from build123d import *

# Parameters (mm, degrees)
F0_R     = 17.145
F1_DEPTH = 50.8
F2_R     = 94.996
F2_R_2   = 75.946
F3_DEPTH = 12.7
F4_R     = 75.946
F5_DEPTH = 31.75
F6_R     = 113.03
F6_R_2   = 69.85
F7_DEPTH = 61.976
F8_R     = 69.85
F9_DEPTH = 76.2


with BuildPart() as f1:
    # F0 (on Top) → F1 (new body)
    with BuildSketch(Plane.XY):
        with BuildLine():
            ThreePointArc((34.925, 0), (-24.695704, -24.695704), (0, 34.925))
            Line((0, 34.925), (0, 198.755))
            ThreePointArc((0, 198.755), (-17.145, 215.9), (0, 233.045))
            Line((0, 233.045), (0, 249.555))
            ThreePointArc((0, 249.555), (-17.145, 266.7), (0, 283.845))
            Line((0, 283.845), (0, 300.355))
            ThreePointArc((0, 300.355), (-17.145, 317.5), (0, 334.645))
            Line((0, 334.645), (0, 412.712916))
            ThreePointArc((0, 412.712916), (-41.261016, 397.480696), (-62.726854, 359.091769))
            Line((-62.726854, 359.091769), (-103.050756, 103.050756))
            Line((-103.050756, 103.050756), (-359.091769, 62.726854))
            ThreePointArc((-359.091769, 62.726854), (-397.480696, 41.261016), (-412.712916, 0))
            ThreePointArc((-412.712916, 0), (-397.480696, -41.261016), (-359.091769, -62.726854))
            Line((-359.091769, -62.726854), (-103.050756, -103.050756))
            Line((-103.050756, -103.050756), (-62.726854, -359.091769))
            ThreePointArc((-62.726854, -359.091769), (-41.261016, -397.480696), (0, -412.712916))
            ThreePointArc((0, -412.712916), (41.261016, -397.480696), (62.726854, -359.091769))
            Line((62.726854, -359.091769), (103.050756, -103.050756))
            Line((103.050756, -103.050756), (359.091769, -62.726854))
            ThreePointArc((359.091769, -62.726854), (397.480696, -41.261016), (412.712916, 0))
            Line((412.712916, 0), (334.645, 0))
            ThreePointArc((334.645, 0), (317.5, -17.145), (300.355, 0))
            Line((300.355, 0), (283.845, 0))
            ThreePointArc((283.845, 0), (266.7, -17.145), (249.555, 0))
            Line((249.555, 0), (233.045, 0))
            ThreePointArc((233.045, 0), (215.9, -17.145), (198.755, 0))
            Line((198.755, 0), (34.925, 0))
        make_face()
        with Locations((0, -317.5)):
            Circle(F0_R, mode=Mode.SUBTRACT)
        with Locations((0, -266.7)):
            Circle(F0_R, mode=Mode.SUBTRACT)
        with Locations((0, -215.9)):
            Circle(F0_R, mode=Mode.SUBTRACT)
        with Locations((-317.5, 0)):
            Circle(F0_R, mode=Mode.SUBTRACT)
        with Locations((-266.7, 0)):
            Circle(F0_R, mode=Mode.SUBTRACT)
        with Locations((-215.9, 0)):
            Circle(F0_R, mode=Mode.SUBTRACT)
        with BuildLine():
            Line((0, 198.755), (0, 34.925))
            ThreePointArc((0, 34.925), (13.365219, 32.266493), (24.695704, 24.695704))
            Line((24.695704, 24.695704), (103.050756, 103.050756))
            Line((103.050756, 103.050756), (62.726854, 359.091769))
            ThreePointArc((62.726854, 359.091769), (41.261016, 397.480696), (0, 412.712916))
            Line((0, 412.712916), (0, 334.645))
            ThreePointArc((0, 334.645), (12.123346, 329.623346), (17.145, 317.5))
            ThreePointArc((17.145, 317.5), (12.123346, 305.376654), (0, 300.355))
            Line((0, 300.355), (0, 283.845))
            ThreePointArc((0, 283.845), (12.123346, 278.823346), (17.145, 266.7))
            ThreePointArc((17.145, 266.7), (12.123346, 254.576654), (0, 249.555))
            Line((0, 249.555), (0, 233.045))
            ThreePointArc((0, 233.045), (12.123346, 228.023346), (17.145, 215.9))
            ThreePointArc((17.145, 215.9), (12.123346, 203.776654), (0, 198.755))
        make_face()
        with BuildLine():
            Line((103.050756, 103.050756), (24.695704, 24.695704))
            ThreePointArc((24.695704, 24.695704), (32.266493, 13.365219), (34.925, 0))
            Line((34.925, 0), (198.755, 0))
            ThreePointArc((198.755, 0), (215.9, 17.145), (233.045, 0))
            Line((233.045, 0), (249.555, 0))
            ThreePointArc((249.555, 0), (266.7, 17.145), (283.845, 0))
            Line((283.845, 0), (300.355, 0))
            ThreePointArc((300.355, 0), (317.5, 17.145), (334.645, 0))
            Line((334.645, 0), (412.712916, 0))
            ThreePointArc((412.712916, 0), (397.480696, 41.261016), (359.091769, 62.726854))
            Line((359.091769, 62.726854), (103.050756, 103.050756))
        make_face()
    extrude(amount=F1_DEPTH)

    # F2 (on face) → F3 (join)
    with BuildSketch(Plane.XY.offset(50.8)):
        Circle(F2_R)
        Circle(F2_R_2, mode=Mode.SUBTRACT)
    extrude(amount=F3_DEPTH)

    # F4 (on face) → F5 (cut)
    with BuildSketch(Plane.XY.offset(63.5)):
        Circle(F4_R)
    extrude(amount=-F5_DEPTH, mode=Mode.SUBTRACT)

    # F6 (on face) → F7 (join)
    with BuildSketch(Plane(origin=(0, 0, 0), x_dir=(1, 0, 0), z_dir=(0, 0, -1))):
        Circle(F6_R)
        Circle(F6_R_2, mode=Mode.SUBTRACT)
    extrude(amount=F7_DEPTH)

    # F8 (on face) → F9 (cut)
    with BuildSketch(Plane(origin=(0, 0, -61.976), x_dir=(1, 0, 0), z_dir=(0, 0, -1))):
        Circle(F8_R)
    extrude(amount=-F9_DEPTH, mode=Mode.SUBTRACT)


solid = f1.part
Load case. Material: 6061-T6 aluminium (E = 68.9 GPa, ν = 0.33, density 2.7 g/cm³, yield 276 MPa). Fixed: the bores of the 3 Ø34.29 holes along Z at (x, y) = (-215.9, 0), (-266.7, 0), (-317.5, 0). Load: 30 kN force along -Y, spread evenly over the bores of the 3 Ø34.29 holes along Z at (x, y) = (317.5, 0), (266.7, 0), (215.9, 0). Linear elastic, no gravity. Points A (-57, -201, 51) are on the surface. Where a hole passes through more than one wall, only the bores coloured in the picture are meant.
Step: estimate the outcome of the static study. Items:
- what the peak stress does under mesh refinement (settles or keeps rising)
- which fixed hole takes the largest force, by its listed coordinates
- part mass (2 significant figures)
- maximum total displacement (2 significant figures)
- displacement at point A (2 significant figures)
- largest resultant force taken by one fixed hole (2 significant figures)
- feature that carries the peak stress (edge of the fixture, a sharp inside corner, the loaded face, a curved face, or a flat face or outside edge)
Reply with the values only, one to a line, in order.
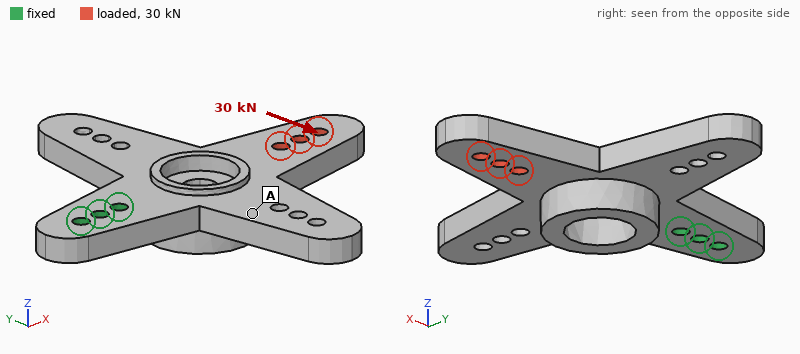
keeps rising
(-215.9, 0)
33 kg
1.3 mm
0.48 mm
140 kN
edge of the fixture
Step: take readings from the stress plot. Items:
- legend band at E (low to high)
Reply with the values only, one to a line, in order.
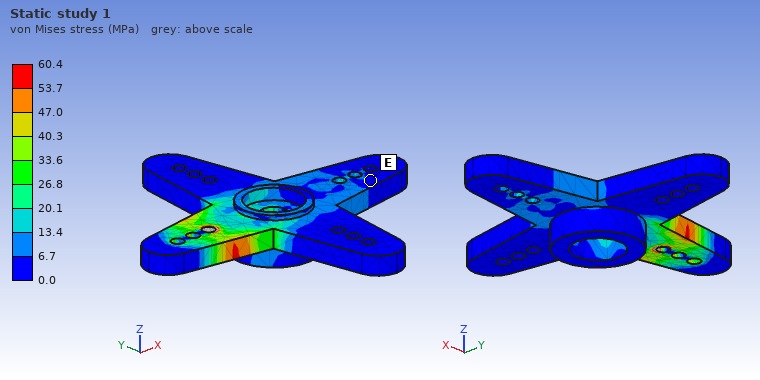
0.0 to 6.7 MPa
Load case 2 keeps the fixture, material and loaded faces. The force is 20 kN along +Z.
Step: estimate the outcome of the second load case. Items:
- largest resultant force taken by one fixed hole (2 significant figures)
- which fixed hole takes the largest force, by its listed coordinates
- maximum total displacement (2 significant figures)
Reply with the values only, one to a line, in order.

67 kN
(-215.9, 0)
6.0 mm
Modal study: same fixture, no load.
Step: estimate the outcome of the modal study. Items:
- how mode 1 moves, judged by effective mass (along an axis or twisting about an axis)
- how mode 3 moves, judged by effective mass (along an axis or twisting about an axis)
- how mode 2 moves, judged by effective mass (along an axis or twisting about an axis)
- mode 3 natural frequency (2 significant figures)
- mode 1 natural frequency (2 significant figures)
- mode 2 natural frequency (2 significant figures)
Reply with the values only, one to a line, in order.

along Z
along Y
twisting about X
250 Hz
120 Hz
190 Hz
